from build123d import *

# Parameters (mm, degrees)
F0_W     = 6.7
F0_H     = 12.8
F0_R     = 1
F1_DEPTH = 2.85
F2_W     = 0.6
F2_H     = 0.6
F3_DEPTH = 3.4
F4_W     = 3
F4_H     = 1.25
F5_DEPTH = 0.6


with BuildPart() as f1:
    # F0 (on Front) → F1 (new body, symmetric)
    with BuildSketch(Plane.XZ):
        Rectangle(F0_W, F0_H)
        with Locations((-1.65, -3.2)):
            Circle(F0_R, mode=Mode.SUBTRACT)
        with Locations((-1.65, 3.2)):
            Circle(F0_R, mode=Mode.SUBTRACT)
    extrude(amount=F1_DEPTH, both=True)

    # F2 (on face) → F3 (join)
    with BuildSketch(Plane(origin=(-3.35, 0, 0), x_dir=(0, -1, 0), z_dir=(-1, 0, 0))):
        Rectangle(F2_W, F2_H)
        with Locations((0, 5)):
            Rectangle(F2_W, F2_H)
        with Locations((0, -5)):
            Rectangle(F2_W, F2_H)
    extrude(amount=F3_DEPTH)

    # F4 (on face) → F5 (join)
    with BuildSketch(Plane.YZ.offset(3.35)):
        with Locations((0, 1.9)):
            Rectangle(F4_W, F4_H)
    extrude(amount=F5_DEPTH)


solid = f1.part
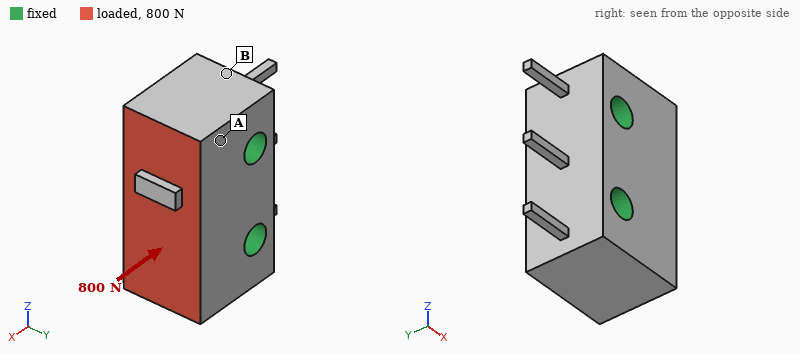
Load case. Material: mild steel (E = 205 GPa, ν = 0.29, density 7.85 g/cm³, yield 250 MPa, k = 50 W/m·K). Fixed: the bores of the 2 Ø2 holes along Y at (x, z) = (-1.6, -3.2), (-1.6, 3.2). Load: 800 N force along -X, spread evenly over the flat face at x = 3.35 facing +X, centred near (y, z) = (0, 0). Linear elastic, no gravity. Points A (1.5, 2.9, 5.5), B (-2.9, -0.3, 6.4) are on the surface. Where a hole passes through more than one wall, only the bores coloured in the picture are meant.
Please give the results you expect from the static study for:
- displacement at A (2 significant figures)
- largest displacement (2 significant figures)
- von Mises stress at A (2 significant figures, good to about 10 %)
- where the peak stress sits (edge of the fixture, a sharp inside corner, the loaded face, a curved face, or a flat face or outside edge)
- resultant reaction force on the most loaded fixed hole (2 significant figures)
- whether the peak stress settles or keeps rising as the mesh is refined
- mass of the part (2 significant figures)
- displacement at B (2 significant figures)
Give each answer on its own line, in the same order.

0.28 µm
0.42 µm
11 MPa
edge of the fixture
410 N
keeps rising
3.6 g
0.18 µm
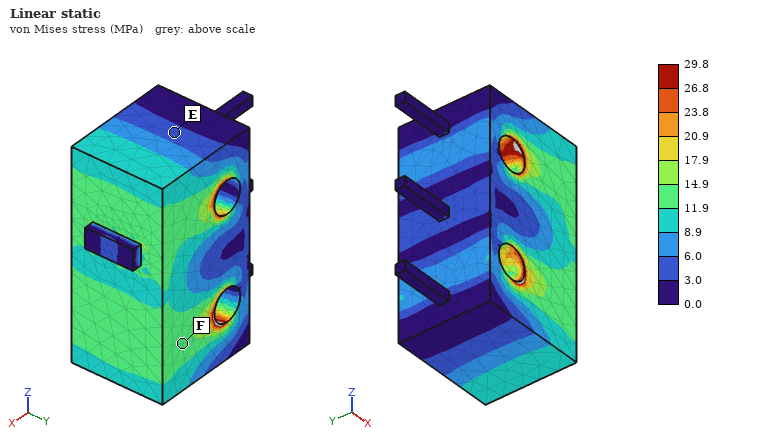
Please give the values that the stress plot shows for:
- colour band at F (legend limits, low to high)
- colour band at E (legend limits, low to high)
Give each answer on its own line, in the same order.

11.9 to 14.9 MPa
3.0 to 6.0 MPa
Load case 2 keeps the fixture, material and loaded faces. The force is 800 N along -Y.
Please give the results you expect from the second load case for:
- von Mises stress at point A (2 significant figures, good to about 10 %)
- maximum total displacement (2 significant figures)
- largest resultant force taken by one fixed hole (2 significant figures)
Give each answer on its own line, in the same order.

22 MPa
2.0 µm
410 N
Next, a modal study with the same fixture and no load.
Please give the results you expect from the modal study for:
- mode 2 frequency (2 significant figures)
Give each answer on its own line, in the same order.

39 kHz
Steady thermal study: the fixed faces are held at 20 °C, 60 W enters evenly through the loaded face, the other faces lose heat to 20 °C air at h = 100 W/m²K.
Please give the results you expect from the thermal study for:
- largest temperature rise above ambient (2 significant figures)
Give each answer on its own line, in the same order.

82 K
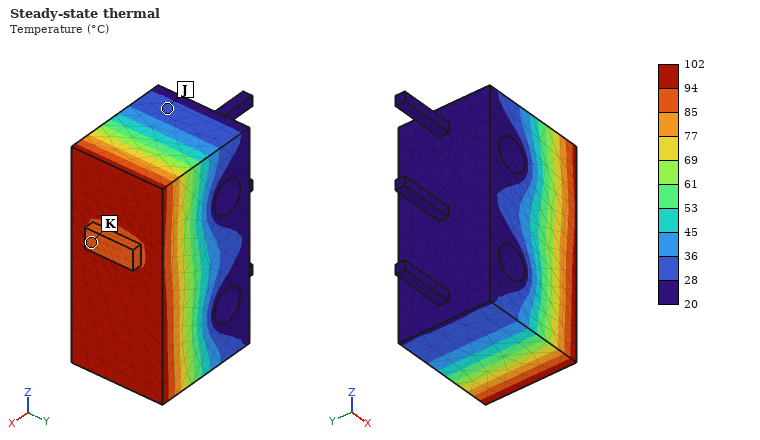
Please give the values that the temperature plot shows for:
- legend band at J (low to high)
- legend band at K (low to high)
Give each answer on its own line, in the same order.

28 to 36 °C
85 to 94 °C
